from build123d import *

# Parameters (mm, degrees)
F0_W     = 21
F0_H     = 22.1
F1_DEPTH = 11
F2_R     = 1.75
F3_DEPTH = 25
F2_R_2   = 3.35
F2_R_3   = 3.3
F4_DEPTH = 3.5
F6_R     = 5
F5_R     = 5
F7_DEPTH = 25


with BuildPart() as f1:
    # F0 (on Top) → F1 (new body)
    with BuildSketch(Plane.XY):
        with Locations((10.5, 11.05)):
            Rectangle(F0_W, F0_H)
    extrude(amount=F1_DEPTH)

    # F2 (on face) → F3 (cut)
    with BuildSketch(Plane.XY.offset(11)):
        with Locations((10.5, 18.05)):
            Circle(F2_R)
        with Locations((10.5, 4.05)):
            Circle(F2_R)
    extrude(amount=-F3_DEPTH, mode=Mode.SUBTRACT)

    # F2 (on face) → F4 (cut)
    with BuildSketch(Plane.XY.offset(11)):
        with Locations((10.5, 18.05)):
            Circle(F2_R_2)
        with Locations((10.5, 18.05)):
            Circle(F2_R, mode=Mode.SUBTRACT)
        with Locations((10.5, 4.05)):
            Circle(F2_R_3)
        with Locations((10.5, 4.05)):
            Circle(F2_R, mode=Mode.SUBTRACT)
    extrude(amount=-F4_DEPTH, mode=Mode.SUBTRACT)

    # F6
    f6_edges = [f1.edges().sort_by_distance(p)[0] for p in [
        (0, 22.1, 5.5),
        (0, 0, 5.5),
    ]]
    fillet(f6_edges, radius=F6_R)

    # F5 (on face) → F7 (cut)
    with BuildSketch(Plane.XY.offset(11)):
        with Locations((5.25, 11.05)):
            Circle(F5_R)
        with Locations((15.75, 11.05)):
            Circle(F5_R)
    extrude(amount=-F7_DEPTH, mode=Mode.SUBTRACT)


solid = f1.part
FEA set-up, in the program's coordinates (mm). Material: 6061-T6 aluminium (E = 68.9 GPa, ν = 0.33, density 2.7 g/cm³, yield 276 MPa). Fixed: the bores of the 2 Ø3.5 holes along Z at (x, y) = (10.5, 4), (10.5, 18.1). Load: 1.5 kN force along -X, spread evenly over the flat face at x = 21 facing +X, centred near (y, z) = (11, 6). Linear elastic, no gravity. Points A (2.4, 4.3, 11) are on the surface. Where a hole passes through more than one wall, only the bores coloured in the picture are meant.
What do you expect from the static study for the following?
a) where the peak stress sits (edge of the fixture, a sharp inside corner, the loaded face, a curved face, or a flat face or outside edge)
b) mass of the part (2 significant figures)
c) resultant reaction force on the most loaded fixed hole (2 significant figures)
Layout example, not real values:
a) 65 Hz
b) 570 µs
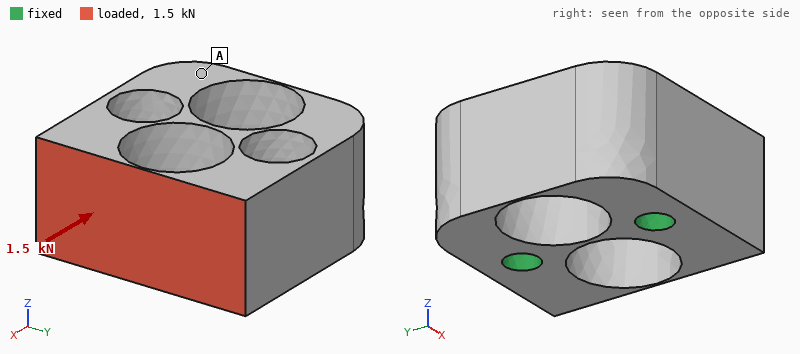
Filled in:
a) the loaded face
b) 7.8 g
c) 780 N
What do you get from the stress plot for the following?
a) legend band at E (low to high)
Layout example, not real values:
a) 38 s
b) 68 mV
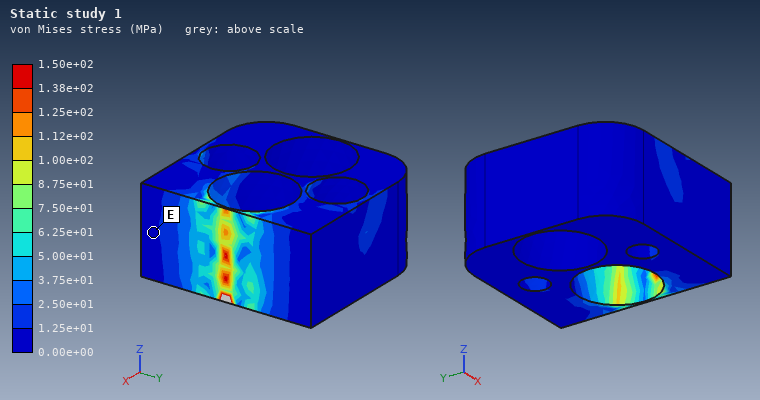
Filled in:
a) 0.00e+00 to 1.25e+01 MPa
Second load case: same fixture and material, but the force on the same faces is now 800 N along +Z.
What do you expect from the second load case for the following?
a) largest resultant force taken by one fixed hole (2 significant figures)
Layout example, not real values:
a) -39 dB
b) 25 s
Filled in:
a) 400 N
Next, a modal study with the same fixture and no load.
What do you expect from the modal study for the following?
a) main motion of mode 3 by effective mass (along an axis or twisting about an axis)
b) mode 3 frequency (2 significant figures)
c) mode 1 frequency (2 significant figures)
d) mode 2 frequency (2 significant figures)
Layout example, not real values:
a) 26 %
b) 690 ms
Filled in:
a) along Y
b) 39 kHz
c) 30 kHz
d) 35 kHz
